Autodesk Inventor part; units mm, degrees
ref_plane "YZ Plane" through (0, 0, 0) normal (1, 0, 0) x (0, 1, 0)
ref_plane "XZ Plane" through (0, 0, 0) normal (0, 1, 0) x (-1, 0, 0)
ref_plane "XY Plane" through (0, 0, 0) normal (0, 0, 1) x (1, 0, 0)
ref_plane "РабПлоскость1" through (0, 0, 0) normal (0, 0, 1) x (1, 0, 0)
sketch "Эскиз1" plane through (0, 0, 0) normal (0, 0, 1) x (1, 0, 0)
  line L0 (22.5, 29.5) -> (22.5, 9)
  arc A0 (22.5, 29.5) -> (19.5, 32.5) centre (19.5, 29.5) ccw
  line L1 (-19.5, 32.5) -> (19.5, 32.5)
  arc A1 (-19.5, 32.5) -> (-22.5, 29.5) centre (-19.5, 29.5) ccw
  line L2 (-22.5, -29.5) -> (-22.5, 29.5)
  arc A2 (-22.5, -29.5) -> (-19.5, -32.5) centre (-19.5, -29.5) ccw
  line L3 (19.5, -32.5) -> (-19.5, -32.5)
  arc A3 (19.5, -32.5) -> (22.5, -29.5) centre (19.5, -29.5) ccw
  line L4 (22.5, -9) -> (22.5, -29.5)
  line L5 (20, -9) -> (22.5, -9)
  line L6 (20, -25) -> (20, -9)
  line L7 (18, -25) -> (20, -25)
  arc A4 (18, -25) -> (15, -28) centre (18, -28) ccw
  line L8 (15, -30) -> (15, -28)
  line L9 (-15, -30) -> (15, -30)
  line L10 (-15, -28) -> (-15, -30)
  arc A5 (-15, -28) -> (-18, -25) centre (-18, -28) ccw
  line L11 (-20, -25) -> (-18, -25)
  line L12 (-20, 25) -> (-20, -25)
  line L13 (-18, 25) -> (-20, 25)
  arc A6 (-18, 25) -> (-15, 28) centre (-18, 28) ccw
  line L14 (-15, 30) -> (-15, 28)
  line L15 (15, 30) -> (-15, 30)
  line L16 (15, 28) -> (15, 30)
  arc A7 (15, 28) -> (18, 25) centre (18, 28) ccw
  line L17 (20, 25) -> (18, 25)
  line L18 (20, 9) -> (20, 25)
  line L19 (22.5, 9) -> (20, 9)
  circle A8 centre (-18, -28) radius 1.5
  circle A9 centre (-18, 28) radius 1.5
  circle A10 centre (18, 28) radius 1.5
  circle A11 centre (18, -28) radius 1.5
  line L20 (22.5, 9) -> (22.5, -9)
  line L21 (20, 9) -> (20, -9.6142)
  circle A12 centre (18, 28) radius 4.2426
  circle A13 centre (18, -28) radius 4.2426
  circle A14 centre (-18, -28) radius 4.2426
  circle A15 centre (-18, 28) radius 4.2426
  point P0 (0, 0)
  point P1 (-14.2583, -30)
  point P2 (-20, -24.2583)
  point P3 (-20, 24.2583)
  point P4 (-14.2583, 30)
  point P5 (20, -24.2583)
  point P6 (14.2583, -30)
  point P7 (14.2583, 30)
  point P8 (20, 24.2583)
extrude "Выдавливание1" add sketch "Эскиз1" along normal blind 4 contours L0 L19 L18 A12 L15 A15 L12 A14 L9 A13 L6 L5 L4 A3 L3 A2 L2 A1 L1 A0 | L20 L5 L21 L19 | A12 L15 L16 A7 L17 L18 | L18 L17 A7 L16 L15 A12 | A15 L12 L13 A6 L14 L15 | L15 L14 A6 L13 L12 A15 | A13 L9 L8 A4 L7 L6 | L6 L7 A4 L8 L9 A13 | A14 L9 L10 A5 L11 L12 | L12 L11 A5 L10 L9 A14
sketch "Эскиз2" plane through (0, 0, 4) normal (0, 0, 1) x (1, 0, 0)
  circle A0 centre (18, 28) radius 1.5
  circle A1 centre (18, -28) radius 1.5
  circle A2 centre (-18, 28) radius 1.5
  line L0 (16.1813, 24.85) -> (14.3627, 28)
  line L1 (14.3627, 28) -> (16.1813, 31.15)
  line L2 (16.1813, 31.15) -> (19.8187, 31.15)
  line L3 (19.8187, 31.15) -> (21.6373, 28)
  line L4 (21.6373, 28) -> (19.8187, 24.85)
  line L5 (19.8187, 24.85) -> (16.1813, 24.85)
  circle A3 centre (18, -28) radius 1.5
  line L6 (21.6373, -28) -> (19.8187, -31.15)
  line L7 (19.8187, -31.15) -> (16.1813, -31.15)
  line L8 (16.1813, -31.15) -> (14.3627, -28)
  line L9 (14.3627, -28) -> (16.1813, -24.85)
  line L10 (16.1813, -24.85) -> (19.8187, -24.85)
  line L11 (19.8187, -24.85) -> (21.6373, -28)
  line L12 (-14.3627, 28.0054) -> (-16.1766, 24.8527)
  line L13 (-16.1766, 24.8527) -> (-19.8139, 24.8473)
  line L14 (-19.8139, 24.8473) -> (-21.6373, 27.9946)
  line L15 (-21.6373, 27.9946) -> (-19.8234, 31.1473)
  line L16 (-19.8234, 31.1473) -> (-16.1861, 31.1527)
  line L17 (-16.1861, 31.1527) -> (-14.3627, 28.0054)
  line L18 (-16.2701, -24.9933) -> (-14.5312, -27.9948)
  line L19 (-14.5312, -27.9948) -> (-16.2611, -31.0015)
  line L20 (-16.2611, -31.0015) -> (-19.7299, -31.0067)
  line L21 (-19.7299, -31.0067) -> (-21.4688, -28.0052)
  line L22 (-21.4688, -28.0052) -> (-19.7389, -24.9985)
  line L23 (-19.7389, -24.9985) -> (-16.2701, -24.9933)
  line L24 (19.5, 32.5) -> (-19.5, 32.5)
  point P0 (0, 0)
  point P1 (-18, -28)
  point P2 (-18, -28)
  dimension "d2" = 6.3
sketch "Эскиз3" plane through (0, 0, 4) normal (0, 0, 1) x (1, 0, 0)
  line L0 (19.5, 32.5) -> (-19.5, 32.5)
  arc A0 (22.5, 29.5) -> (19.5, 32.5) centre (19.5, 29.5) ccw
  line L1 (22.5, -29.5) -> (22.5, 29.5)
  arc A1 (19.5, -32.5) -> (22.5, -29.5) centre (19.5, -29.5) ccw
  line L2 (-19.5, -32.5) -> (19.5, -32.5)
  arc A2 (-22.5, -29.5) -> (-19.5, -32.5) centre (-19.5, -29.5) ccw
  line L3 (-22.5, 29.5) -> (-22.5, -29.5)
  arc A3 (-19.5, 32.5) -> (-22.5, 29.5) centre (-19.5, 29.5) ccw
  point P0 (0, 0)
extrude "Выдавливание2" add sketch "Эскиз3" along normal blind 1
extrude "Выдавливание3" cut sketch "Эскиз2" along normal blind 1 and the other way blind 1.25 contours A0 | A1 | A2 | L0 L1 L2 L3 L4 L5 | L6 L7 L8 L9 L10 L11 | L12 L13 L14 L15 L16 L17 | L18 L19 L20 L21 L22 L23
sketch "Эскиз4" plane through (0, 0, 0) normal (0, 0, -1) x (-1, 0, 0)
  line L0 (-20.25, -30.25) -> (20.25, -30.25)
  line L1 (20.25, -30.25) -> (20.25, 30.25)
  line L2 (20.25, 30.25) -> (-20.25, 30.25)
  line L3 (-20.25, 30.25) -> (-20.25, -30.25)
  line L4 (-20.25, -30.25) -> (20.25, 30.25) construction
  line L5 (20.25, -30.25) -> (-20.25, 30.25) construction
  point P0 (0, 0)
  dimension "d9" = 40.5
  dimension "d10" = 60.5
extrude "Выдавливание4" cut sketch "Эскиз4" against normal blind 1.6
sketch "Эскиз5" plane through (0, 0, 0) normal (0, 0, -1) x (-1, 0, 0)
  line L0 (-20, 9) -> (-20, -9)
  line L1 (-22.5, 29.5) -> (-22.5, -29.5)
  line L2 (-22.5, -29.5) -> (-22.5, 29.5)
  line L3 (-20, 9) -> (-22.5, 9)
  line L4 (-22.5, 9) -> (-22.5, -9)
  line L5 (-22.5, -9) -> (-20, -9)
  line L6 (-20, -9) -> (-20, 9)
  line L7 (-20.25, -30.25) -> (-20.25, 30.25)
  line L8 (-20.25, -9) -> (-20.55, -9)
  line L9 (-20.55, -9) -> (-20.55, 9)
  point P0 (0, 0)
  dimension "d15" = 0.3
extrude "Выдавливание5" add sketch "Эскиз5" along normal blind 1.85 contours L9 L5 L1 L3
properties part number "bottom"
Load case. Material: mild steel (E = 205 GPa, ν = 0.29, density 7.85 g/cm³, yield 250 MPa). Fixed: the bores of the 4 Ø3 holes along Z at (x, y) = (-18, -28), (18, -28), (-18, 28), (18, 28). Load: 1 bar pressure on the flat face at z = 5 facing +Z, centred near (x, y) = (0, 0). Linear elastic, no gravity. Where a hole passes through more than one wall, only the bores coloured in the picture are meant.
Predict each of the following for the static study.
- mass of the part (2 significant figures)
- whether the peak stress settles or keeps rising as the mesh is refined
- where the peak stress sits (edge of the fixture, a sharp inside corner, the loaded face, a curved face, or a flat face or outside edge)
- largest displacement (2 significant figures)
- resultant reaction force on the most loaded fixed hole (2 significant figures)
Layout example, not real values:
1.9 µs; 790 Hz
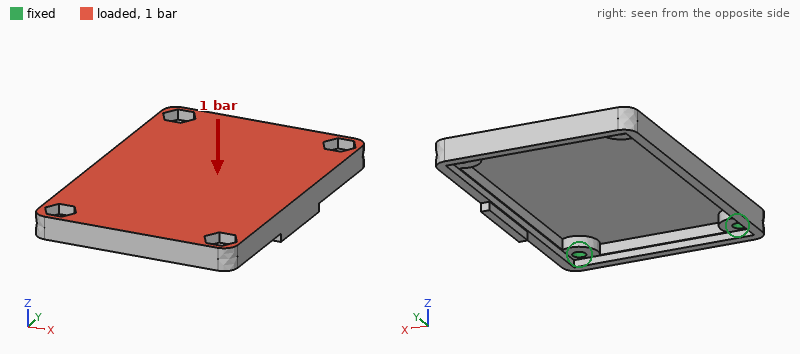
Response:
39 g; keeps rising; edge of the fixture; 54 µm; 140 N
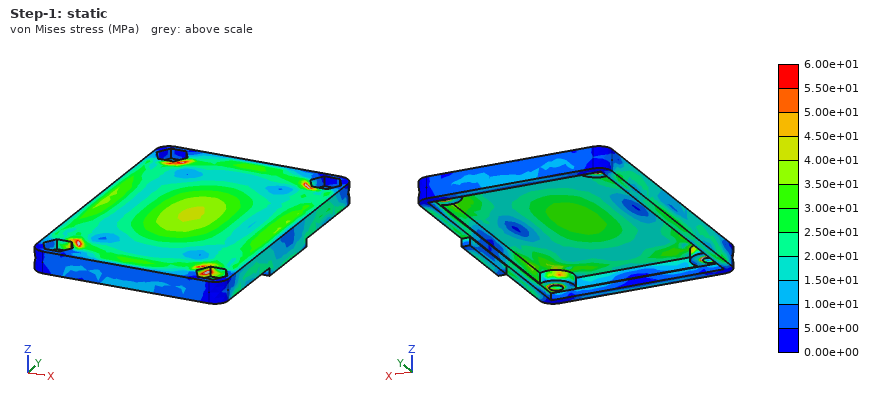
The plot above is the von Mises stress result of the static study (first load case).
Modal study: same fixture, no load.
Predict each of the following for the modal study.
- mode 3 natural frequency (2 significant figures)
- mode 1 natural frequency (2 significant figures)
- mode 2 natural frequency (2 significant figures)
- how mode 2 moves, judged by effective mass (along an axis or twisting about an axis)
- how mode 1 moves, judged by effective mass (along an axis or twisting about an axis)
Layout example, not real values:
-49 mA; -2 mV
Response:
5700 Hz; 3100 Hz; 5300 Hz; twisting about Y; along Z
